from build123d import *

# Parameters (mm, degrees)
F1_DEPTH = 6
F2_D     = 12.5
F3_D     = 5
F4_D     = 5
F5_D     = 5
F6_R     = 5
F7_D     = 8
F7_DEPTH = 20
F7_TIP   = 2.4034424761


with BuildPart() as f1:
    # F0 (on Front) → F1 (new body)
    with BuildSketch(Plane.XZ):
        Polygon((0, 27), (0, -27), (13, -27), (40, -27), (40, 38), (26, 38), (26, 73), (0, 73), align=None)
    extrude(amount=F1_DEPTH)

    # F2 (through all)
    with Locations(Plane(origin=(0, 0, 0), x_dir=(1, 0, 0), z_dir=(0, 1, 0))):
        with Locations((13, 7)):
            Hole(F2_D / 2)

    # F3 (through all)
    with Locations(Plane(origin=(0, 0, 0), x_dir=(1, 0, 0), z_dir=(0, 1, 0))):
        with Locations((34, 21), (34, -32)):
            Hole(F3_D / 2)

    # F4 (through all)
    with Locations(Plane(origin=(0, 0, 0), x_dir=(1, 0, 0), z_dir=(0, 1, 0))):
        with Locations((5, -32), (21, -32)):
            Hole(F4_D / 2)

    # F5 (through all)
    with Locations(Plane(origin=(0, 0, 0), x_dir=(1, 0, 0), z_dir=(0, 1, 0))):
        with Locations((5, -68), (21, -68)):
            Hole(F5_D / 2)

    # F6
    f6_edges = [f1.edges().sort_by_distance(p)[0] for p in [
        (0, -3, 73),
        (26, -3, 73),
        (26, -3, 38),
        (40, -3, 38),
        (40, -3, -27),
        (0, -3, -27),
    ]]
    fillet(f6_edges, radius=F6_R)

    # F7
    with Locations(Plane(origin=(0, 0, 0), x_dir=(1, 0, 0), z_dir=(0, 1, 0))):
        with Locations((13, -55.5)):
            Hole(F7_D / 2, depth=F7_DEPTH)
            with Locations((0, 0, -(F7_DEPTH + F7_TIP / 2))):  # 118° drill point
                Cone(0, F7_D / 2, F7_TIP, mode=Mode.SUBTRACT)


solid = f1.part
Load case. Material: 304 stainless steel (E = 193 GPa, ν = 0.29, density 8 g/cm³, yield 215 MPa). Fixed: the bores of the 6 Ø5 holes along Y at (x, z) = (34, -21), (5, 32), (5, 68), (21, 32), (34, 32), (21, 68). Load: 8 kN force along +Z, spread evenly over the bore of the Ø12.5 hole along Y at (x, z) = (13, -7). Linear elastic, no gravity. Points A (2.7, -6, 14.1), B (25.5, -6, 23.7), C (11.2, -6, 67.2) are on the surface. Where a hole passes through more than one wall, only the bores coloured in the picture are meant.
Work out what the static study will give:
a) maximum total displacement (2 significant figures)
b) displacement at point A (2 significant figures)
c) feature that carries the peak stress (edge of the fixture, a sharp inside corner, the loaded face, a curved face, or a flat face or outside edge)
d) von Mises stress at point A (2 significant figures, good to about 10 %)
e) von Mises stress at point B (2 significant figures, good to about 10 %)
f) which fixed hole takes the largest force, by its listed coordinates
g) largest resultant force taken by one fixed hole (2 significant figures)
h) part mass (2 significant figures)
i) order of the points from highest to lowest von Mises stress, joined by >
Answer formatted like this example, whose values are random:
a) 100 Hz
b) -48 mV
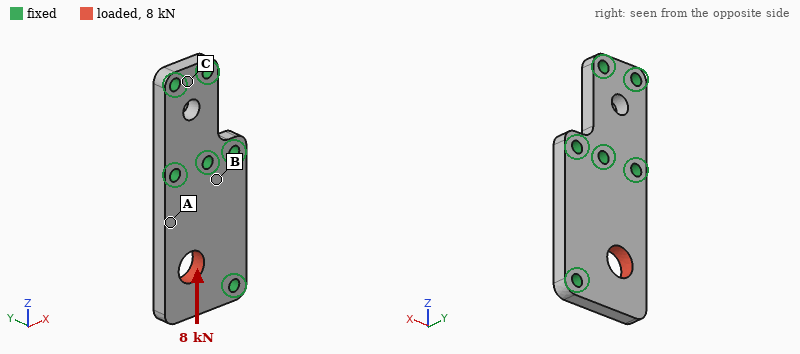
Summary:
a) 10 µm
b) 3.2 µm
c) edge of the fixture
d) 43 MPa
e) 21 MPa
f) (34, -21)
g) 2.8 kN
h) 150 g
i) A > B > C
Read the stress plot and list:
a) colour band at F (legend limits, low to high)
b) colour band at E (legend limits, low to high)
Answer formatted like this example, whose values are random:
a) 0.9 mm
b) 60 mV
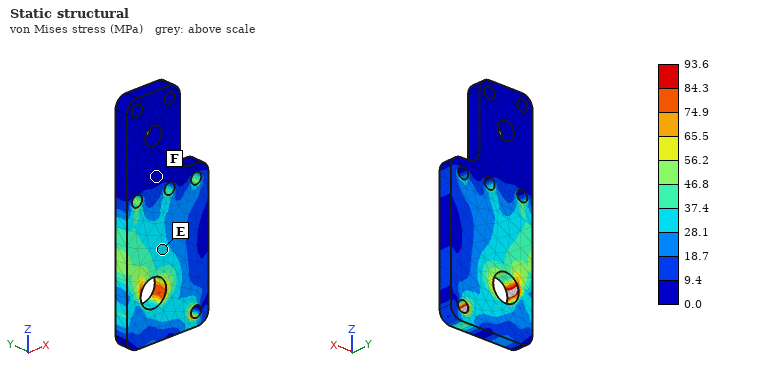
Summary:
a) 0.0 to 9.4 MPa
b) 28.1 to 37.4 MPa
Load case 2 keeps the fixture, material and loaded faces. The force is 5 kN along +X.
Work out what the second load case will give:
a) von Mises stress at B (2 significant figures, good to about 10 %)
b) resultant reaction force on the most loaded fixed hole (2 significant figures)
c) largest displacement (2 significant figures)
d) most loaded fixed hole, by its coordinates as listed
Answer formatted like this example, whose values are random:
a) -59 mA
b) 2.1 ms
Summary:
a) 19 MPa
b) 3.3 kN
c) 7.1 µm
d) (34, -21)
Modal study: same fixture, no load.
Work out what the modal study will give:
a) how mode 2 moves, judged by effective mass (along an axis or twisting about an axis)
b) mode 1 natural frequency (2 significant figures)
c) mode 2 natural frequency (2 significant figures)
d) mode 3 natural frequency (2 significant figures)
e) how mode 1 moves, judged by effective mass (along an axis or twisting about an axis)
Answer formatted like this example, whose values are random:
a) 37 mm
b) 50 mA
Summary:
a) along Y
b) 5100 Hz
c) 9900 Hz
d) 13 kHz
e) along Y
